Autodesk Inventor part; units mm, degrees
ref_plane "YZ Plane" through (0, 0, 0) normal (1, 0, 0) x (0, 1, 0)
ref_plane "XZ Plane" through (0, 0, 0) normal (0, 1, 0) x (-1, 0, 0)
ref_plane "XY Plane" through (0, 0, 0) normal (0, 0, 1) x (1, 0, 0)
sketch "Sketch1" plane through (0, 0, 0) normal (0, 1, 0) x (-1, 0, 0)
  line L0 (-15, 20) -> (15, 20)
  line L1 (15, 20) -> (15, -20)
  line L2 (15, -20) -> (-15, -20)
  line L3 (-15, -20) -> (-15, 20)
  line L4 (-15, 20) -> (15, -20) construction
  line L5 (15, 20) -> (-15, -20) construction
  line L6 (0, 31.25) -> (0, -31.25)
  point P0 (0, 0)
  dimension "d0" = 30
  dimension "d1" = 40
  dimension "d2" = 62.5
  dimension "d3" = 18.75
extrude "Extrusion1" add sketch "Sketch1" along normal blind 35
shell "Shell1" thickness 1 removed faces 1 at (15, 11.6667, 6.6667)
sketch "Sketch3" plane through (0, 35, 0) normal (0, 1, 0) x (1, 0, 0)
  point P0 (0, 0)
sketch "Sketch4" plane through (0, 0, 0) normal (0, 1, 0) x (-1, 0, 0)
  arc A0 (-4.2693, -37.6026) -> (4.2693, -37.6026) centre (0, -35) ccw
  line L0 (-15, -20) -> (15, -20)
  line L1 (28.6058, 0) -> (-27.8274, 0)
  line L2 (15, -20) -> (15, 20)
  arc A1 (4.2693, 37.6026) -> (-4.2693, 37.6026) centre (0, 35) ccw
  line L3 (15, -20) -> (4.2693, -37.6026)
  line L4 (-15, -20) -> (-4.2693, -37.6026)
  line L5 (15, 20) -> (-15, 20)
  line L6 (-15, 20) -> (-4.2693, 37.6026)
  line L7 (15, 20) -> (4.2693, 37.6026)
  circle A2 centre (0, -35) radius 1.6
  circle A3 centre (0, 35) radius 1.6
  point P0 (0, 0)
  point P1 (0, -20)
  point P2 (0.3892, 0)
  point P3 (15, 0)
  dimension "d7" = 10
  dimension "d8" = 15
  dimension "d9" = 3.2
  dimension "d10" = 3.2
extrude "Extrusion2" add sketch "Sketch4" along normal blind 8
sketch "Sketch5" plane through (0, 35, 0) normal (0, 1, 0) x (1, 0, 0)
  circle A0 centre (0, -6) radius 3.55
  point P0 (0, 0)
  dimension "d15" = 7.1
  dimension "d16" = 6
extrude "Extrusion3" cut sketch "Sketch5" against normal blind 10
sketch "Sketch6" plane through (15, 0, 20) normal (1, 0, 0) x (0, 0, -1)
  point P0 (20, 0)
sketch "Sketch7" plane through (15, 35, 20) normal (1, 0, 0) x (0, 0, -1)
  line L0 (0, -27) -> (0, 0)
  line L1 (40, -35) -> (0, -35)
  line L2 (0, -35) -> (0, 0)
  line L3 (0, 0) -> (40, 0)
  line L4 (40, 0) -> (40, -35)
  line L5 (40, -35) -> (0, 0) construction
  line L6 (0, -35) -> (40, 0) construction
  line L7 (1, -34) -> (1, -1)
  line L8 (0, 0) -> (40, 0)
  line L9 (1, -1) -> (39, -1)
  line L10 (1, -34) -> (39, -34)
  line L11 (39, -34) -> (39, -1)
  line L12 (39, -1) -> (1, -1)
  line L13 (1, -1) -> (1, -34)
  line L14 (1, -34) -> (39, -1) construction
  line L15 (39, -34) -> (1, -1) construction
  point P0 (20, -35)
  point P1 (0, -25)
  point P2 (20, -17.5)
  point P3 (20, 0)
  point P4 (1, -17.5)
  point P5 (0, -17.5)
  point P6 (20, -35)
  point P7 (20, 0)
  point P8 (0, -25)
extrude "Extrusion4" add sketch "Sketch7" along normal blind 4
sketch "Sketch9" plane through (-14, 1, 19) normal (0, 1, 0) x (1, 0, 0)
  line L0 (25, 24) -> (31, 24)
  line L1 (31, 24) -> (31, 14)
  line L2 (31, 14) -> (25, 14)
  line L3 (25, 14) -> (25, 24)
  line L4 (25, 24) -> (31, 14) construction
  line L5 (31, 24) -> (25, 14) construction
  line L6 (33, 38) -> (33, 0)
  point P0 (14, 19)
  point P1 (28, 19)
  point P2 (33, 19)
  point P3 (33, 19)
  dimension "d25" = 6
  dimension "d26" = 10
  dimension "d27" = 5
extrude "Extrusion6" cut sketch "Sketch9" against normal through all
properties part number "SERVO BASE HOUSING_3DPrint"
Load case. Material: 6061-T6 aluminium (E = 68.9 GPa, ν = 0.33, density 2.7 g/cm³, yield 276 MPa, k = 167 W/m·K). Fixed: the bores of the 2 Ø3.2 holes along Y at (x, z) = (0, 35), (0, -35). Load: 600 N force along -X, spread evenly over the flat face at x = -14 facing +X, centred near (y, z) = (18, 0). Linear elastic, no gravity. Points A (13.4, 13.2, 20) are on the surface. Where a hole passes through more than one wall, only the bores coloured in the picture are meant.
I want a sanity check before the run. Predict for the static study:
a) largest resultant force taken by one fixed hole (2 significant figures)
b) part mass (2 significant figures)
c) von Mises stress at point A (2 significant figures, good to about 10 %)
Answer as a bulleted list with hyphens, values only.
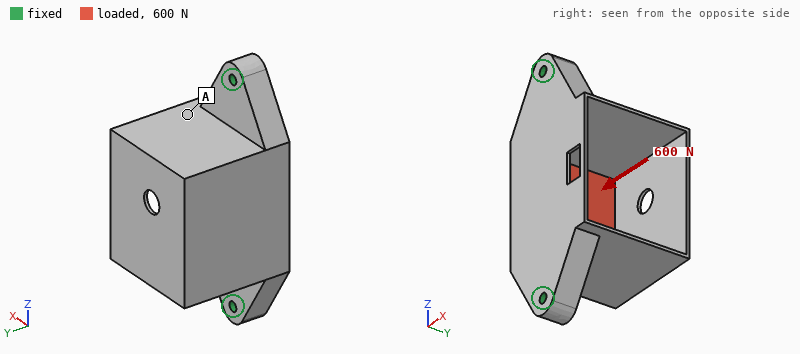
- 320 N
- 31 g
- 11 MPa
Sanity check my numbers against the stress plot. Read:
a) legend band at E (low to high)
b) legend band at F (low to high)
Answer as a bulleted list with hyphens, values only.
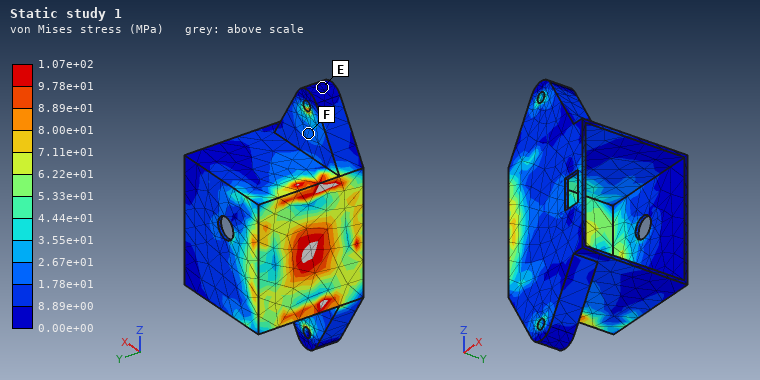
- 0.00e+00 to 8.89e+00 MPa
- 1.78e+01 to 2.67e+01 MPa
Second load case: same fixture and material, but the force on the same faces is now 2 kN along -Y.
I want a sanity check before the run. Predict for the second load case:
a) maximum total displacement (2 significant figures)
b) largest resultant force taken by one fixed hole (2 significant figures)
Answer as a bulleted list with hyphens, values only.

- 0.17 mm
- 1.0 kN
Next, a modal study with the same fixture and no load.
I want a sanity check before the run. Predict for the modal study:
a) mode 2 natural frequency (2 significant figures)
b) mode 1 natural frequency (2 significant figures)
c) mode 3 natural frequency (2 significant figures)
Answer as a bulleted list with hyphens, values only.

- 3000 Hz
- 2900 Hz
- 3900 Hz
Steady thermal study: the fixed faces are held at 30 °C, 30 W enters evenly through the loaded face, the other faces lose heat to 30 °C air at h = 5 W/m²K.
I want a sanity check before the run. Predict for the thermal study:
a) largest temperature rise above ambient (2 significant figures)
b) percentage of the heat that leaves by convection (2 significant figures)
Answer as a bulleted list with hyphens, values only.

- 49 K
- 4.7 %
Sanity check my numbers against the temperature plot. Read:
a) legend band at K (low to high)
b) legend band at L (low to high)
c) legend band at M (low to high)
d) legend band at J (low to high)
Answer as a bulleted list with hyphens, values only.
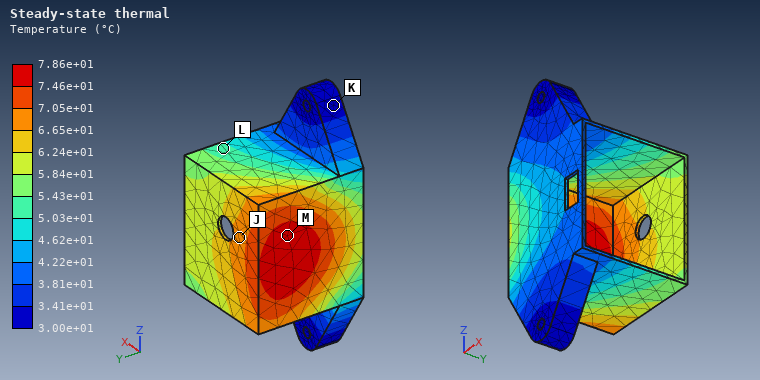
- 3.00e+01 to 3.41e+01 °C
- 5.03e+01 to 5.43e+01 °C
- 7.46e+01 to 7.86e+01 °C
- 6.65e+01 to 7.05e+01 °C
